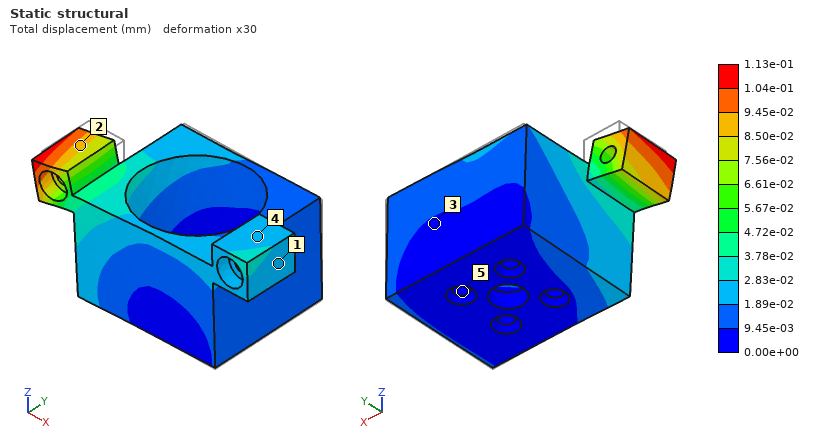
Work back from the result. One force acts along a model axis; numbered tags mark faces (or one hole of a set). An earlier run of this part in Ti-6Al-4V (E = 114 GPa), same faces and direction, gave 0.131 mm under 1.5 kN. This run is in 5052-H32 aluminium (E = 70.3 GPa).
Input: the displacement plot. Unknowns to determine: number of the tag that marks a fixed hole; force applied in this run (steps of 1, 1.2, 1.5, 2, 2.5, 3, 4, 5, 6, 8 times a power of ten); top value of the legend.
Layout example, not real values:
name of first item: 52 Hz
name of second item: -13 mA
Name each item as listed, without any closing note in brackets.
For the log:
number of the tag that marks a fixed hole: 5
force applied in this run: 800 N
top value of the legend: 1.13e-01 mm
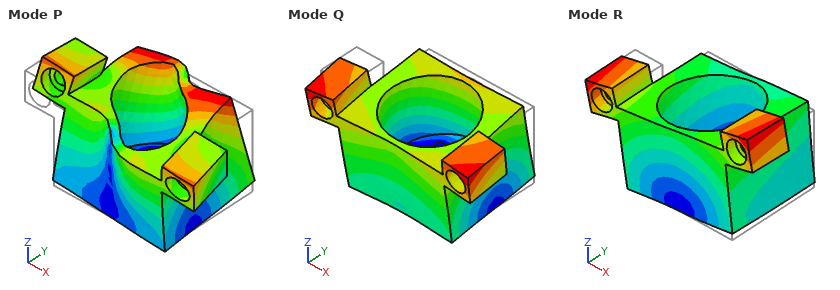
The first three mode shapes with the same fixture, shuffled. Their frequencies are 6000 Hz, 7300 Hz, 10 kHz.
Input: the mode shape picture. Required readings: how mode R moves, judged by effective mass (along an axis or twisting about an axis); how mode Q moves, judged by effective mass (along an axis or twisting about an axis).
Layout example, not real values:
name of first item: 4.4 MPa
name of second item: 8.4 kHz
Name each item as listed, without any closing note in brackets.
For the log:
how mode R moves, judged by effective mass: along X
how mode Q moves, judged by effective mass: along Y
